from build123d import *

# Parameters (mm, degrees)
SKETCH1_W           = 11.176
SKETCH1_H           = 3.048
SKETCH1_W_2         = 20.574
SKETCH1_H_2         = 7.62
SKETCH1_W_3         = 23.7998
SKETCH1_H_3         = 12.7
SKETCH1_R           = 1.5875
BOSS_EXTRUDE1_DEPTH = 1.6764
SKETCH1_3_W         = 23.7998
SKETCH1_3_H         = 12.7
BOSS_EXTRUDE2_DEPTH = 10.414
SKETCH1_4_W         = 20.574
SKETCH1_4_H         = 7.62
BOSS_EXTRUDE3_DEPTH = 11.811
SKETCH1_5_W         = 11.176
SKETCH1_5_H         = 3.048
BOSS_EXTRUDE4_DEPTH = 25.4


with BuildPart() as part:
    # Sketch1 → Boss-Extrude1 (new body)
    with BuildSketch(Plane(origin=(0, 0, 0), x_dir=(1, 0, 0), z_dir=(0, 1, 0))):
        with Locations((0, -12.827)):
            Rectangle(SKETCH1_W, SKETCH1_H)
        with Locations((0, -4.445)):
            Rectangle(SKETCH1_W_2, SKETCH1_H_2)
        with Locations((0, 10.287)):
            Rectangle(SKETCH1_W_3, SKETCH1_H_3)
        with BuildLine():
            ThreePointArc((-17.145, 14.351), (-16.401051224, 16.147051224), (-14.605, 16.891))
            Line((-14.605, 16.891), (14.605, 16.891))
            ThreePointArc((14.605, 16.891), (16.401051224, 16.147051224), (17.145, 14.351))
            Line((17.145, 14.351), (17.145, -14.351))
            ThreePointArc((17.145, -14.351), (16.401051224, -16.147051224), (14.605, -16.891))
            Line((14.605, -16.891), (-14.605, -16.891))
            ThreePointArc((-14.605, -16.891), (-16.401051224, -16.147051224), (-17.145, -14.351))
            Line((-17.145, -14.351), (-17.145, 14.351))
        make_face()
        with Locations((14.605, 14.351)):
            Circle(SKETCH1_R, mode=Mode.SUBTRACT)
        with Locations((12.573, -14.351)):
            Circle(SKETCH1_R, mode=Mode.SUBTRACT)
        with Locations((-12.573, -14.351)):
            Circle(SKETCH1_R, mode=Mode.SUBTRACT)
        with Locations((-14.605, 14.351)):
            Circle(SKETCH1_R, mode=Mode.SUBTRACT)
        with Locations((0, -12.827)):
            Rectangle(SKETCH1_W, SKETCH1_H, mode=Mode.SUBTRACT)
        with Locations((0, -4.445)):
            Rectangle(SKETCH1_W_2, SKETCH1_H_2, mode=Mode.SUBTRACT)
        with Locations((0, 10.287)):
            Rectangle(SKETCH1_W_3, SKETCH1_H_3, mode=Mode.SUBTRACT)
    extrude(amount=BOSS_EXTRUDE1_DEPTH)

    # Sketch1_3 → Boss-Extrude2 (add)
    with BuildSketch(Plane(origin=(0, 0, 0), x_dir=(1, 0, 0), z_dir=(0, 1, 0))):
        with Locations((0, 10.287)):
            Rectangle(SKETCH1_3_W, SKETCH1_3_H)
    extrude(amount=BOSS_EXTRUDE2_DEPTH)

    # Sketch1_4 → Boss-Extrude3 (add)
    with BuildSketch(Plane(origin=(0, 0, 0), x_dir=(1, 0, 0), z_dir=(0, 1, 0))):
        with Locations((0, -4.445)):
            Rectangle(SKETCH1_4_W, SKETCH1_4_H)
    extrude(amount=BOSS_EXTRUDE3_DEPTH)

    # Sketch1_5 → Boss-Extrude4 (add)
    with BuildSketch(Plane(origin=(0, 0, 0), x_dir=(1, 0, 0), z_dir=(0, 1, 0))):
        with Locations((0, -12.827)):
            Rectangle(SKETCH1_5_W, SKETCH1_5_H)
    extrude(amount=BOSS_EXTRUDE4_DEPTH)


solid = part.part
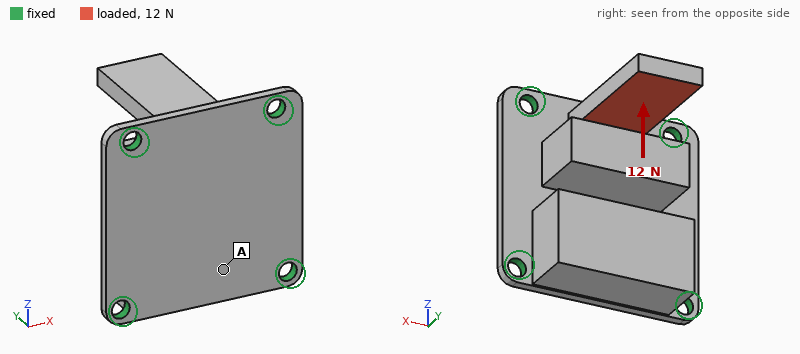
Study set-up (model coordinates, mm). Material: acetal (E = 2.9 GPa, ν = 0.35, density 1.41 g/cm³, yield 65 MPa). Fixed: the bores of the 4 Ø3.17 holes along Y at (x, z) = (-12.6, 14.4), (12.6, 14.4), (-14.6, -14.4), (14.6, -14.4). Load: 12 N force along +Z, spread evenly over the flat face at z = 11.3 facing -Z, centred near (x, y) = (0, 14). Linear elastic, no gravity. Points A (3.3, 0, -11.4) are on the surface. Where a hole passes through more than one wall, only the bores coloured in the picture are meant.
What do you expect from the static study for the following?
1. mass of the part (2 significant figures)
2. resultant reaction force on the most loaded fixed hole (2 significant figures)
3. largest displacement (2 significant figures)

9.8 g
4.6 N
0.65 mm
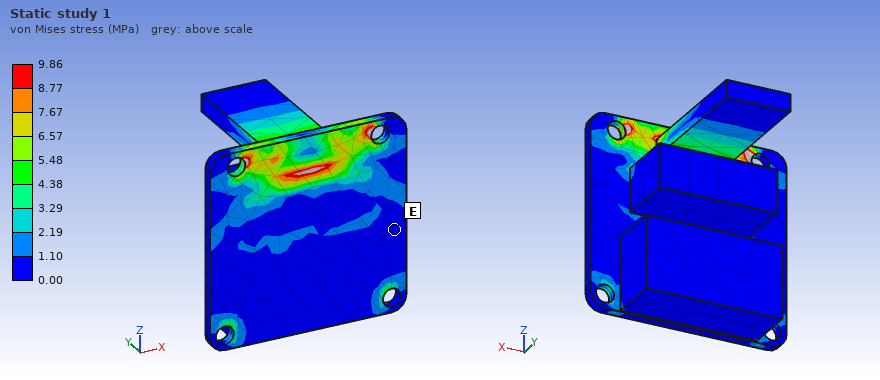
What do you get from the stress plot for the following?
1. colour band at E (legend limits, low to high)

0.00 to 1.10 MPa
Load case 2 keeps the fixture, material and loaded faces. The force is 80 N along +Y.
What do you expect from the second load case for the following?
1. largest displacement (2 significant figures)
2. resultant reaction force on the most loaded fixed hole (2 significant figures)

0.40 mm
39 N
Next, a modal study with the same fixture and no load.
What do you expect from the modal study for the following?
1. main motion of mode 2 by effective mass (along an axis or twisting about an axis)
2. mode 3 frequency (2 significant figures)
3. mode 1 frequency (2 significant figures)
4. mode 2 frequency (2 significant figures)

along Y
2000 Hz
780 Hz
1600 Hz
